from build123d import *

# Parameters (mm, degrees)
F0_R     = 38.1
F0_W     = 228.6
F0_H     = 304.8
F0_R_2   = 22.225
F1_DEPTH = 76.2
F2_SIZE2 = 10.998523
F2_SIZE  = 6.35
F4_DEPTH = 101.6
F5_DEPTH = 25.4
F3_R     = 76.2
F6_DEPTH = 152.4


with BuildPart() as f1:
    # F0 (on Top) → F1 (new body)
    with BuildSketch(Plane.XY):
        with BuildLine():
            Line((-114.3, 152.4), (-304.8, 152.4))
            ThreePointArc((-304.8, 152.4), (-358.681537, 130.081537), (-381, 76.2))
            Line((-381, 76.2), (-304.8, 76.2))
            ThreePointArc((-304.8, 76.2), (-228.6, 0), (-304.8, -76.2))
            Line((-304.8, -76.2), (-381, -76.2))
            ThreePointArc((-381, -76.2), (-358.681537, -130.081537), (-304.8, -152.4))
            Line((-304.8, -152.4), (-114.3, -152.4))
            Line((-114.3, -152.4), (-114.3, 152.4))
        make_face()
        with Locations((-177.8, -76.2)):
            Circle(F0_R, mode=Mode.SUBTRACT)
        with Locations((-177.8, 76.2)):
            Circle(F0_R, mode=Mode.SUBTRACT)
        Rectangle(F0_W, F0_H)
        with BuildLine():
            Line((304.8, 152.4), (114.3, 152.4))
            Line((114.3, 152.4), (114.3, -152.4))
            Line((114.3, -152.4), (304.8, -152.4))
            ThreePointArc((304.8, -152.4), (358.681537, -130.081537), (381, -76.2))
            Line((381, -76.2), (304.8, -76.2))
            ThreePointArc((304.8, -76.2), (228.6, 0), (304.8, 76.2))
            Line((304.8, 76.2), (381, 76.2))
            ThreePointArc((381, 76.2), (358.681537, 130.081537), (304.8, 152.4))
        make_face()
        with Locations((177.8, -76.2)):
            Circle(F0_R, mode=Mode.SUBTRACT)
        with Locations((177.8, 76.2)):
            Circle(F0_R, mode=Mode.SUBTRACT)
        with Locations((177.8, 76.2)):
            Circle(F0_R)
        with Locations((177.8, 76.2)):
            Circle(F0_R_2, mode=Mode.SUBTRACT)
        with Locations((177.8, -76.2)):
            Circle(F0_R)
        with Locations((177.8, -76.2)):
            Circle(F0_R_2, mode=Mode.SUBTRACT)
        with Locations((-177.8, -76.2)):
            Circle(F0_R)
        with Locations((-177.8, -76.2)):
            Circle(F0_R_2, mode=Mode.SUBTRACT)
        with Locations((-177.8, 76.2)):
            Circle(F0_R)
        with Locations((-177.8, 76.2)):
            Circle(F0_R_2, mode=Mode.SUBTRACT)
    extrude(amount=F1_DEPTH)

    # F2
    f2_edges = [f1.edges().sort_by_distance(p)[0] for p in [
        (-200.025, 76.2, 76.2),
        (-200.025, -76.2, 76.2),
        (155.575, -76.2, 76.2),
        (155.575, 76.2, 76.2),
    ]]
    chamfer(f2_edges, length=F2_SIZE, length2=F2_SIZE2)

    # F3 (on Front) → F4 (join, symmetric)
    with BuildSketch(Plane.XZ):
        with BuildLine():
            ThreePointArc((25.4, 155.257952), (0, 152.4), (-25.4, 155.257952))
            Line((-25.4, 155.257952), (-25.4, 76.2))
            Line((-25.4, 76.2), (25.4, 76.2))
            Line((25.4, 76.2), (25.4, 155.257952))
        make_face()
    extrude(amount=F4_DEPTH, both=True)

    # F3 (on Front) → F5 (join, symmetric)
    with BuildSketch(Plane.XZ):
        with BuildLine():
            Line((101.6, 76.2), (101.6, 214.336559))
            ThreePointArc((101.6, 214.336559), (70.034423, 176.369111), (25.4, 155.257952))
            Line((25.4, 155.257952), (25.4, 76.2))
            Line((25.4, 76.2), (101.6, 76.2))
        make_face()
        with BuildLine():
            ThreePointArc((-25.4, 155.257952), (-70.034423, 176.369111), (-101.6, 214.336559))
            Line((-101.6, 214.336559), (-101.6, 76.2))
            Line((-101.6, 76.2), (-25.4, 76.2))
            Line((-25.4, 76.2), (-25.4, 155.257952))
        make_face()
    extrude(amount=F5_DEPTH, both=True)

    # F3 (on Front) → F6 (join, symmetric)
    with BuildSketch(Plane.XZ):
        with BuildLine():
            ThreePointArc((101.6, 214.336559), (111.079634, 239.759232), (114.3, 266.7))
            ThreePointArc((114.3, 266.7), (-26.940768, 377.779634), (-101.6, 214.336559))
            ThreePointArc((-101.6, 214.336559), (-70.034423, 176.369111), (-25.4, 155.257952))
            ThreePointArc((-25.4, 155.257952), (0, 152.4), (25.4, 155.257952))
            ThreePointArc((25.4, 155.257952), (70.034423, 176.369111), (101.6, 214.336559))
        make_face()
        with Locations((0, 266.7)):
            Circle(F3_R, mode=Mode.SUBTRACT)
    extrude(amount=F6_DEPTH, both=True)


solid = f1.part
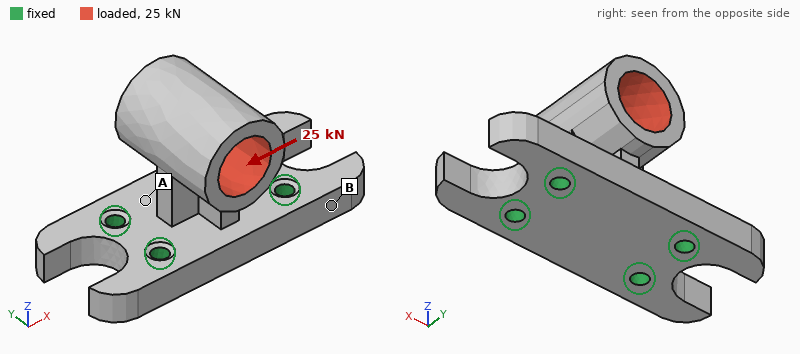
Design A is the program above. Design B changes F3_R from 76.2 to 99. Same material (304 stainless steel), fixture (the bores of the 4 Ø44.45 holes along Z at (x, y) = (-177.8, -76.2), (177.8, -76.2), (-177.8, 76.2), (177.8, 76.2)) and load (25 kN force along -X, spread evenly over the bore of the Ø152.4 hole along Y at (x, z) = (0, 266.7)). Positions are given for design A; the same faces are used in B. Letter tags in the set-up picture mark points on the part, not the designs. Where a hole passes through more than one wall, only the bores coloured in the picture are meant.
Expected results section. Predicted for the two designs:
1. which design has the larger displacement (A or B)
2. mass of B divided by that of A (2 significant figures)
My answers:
B
0.83
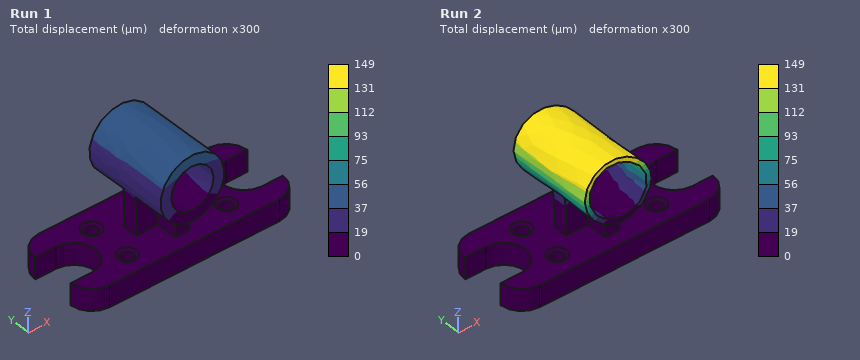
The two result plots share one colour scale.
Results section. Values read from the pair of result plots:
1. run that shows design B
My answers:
Run 2
